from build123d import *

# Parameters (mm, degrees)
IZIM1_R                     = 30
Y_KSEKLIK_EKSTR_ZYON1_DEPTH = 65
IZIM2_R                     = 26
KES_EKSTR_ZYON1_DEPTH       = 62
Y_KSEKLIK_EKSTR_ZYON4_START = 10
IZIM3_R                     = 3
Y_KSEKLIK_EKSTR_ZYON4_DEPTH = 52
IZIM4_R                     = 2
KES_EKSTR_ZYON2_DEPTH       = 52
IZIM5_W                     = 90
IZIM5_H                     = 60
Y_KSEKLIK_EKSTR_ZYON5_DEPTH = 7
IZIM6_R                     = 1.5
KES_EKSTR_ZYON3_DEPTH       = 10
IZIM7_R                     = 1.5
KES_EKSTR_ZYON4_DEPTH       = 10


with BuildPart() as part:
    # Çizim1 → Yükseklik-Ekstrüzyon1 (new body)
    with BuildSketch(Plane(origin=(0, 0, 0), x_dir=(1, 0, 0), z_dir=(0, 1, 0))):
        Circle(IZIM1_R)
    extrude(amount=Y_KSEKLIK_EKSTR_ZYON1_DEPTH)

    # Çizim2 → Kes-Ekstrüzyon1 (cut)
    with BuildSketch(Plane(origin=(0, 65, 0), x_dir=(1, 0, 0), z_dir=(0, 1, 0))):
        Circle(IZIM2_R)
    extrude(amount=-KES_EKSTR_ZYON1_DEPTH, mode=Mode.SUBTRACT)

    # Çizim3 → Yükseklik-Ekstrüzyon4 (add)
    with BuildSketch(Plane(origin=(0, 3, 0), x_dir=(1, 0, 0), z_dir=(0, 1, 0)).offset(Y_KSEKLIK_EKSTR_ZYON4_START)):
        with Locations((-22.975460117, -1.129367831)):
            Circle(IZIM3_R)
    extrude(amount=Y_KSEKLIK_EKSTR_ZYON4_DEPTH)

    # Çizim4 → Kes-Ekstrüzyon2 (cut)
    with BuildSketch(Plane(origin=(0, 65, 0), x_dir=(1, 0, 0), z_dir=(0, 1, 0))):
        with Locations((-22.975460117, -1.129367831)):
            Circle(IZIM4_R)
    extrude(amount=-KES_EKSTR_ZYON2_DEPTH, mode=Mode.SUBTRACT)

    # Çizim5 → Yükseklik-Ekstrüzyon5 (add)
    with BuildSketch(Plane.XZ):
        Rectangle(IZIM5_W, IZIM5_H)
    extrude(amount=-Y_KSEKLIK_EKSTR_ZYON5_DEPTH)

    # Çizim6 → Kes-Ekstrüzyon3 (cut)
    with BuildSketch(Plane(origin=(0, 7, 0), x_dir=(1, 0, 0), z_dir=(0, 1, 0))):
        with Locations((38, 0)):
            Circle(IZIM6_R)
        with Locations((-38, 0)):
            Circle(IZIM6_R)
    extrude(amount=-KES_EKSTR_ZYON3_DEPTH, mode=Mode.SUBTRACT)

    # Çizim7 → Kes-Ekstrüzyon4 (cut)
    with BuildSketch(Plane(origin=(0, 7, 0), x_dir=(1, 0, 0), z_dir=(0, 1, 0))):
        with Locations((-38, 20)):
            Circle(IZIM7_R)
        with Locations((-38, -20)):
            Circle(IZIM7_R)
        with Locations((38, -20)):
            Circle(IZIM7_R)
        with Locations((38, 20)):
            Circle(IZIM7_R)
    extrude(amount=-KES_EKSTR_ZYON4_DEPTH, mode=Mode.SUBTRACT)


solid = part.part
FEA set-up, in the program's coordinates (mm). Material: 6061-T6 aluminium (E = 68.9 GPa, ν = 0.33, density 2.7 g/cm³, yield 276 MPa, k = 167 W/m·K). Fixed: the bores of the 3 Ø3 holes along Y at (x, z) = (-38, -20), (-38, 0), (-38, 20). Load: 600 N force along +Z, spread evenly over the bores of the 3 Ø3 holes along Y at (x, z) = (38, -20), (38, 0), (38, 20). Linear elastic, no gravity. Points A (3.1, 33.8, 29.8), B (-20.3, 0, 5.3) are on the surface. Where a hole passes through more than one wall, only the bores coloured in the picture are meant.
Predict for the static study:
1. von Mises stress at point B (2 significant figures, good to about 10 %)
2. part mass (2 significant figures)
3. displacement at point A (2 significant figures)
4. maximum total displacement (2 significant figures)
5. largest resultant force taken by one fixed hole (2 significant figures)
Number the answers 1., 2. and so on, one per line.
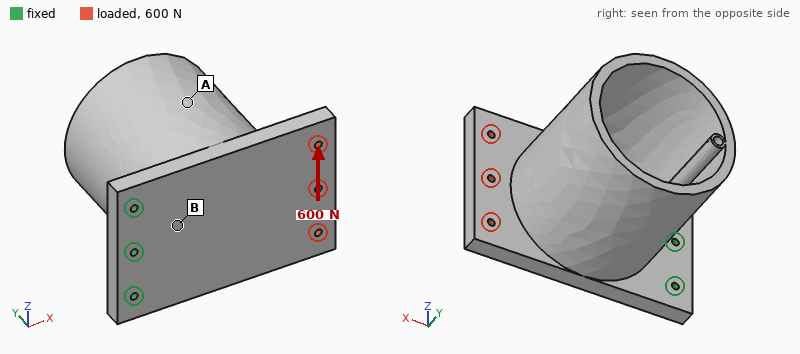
1. 5.0 MPa
2. 210 g
3. 10 µm
4. 21 µm
5. 1.1 kN
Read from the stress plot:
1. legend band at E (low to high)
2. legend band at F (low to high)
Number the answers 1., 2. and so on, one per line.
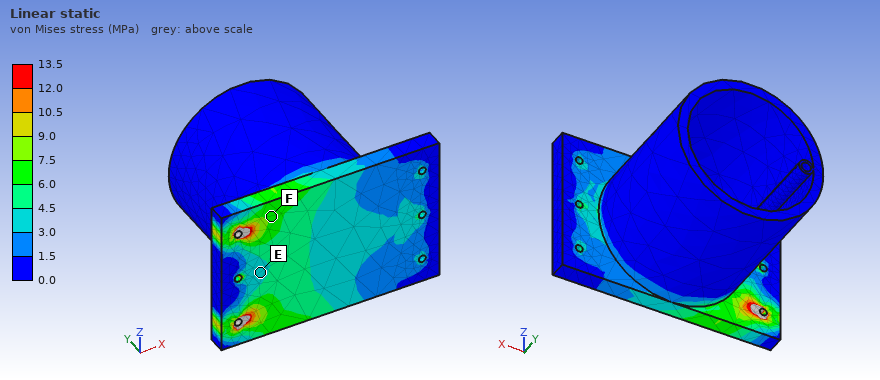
1. 3.0 to 4.5 MPa
2. 6.0 to 7.5 MPa
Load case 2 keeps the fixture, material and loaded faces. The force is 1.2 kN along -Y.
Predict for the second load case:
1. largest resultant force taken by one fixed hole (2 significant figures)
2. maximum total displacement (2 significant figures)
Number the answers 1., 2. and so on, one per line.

1. 770 N
2. 1.2 mm
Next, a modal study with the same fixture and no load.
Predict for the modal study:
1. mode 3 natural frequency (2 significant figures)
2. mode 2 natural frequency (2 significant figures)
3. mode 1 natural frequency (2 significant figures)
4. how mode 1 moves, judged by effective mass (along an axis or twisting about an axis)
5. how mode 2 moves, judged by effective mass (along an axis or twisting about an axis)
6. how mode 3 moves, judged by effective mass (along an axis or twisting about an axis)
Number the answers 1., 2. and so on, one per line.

1. 3700 Hz
2. 1700 Hz
3. 580 Hz
4. along Y
5. along Z
6. along Z
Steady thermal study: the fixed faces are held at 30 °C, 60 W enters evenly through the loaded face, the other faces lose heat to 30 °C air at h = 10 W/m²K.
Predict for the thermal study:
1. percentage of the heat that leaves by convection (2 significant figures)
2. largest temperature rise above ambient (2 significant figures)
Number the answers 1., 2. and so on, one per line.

1. 14 %
2. 53 K
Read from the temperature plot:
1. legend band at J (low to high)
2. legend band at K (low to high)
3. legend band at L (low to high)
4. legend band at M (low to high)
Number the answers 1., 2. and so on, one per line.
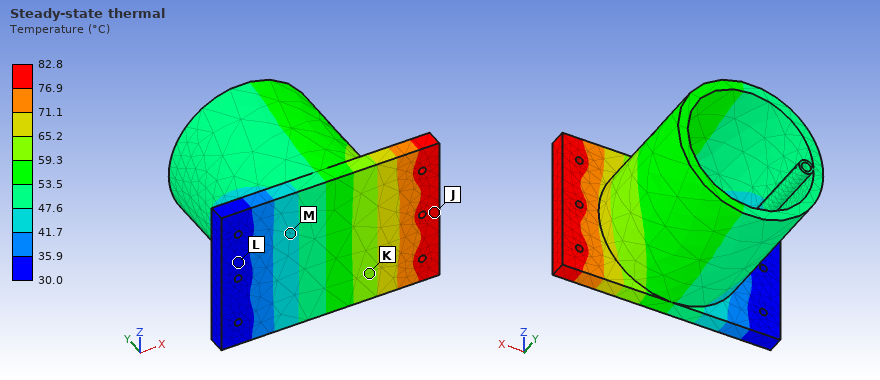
1. 76.9 to 82.8 °C
2. 59.3 to 65.2 °C
3. 30.0 to 35.9 °C
4. 41.7 to 47.6 °C
